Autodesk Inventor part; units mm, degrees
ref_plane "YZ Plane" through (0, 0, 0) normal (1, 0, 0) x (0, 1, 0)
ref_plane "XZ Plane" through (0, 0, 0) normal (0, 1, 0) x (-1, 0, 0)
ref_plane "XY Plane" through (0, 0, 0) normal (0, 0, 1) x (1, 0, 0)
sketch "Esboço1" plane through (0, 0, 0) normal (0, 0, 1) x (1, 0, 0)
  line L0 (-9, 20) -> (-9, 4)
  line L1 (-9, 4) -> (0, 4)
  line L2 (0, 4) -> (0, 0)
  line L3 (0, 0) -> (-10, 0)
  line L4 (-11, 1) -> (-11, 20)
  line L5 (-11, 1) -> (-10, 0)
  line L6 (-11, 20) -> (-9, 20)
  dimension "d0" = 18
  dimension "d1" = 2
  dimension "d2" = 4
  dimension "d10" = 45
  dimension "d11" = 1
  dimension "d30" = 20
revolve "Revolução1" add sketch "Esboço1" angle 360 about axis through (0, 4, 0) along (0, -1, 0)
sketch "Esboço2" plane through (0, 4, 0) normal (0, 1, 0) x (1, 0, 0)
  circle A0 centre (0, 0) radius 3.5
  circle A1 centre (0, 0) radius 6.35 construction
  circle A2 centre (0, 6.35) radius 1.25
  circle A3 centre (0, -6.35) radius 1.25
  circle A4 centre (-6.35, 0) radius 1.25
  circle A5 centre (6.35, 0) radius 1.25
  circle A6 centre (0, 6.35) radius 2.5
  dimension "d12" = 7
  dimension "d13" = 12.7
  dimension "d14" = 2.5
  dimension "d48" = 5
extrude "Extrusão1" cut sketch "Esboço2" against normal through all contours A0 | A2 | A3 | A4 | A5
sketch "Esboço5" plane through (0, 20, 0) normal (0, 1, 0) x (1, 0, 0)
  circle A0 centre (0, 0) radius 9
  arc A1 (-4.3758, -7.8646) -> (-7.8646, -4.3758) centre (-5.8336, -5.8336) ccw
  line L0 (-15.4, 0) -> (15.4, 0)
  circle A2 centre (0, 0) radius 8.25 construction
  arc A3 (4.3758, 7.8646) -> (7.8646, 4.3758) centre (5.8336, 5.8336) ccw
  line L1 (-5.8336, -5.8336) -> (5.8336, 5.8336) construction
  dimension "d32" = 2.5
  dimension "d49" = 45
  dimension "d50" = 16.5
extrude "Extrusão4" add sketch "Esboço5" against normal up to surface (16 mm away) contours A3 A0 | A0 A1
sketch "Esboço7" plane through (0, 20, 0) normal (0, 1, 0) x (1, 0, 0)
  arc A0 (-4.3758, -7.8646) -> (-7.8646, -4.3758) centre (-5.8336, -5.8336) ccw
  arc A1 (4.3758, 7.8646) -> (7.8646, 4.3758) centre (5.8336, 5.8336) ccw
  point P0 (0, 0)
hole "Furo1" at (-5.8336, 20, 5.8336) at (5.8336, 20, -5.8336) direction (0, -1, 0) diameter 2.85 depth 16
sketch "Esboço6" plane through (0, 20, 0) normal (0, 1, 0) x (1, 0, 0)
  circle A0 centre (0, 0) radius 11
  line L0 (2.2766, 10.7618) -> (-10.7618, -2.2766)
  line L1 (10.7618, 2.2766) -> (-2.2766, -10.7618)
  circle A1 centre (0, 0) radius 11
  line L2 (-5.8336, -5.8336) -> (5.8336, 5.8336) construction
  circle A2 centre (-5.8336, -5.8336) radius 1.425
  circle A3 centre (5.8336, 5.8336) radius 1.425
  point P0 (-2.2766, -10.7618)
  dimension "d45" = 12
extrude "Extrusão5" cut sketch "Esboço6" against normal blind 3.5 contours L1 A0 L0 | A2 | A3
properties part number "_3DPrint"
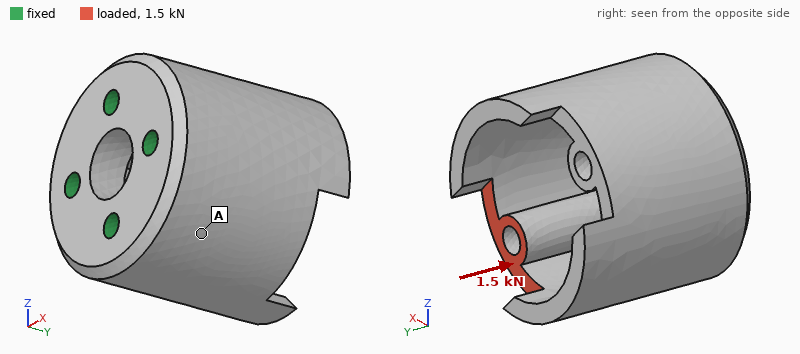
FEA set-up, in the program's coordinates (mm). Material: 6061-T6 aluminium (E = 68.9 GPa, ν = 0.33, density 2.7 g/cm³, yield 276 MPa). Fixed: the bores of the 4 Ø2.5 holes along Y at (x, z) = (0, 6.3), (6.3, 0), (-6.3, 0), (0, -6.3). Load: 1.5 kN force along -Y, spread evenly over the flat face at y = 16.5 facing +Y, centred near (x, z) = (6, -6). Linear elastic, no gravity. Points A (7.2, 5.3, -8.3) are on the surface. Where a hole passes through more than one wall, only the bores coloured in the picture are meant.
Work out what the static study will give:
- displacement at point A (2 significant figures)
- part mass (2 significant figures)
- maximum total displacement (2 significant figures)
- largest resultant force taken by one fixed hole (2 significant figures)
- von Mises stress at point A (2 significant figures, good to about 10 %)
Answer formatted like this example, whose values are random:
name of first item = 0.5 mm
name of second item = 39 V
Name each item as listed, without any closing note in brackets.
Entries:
displacement at point A = 12 µm
part mass = 8.8 g
maximum total displacement = 27 µm
largest resultant force taken by one fixed hole = 850 N
von Mises stress at point A = 25 MPa
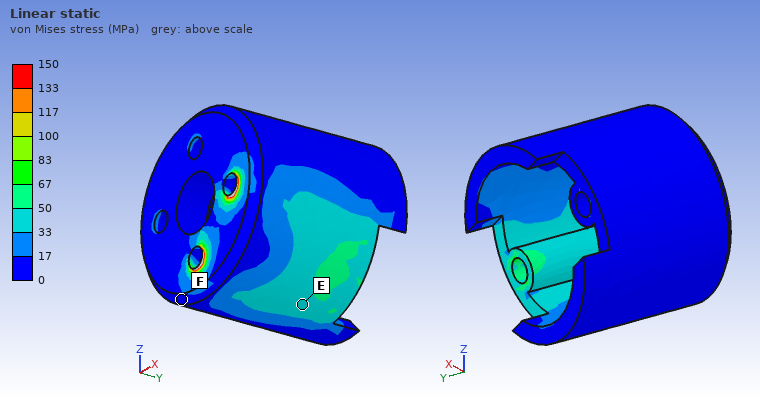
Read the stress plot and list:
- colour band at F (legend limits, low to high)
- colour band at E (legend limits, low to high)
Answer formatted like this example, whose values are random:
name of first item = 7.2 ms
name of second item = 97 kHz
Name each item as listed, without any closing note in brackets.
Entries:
colour band at F = 0 to 17 MPa
colour band at E = 33 to 50 MPa
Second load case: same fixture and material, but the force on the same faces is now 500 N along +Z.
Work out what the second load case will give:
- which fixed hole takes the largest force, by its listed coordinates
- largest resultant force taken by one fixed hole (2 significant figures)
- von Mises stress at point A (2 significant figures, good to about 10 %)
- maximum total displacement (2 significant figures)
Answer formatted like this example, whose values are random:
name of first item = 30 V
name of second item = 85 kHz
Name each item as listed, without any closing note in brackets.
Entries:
which fixed hole takes the largest force, by its listed coordinates = (0, -6.3)
largest resultant force taken by one fixed hole = 490 N
von Mises stress at point A = 23 MPa
maximum total displacement = 38 µm
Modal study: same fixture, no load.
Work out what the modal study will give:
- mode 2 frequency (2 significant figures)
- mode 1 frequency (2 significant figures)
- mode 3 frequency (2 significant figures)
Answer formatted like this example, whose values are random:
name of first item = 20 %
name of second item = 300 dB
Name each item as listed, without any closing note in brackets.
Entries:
mode 2 frequency = 20 kHz
mode 1 frequency = 17 kHz
mode 3 frequency = 20 kHz
